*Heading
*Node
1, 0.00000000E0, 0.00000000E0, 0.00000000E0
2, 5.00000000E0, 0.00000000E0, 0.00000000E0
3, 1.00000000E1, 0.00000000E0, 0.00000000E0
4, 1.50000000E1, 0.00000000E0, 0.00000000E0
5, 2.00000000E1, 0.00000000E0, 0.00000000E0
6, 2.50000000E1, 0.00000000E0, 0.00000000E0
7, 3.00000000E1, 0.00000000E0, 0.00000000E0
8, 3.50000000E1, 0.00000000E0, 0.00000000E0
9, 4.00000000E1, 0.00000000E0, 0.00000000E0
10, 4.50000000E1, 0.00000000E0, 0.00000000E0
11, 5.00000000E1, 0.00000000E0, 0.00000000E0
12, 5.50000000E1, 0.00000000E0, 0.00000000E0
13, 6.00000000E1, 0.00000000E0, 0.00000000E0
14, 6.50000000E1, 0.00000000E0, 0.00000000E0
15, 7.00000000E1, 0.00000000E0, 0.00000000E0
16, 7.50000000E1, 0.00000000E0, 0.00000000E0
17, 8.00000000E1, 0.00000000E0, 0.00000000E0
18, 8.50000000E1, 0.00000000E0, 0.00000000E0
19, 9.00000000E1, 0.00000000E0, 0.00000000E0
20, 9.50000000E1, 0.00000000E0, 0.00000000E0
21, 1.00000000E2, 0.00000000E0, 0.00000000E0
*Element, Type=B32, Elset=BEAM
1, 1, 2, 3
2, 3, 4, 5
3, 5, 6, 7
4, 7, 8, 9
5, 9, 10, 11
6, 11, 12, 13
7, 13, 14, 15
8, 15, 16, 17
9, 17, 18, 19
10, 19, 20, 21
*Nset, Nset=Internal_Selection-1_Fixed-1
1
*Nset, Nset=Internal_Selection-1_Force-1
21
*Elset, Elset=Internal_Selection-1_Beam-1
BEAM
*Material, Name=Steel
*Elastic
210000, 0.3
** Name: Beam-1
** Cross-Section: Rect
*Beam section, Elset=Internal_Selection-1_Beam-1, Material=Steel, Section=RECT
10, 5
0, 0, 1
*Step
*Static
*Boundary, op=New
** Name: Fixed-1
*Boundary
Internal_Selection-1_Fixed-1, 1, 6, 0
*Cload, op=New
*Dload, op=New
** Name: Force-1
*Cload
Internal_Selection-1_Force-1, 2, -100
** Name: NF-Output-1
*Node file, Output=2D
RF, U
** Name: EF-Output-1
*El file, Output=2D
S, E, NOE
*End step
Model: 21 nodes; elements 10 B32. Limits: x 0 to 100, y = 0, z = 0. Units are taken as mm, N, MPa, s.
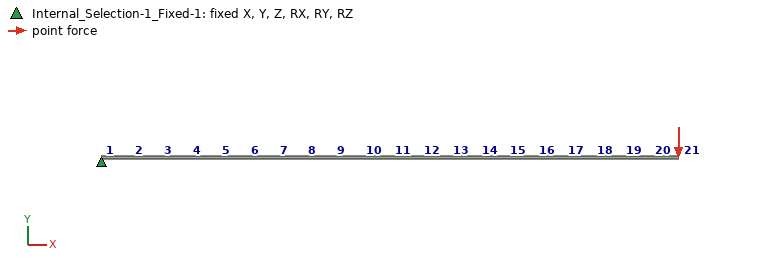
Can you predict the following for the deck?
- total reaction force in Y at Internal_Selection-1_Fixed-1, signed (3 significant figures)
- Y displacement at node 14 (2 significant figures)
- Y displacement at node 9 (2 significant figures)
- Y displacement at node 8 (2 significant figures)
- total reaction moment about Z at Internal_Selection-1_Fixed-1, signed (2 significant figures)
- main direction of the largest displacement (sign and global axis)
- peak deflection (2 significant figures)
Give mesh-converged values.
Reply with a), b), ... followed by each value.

a) 100 N
b) -0.76 mm
c) -0.32 mm
d) -0.25 mm
e) 10000 N·mm
f) -Y
g) 1.5 mm
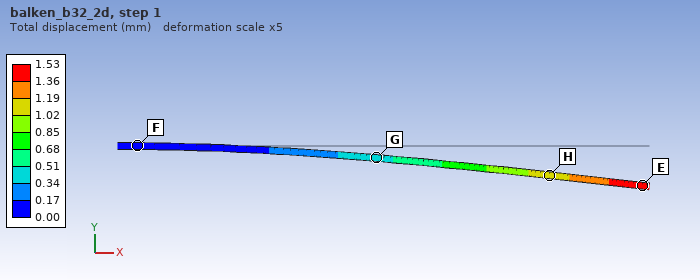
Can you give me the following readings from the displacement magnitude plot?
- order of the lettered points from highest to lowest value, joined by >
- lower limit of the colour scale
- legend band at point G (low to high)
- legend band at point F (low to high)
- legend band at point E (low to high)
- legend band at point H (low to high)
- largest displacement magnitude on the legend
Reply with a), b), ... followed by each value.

a) E > H > G > F
b) 0.00 mm
c) 0.34 to 0.51 mm
d) 0.00 to 0.17 mm
e) 1.36 to 1.53 mm
f) 1.02 to 1.19 mm
g) 1.53 mm
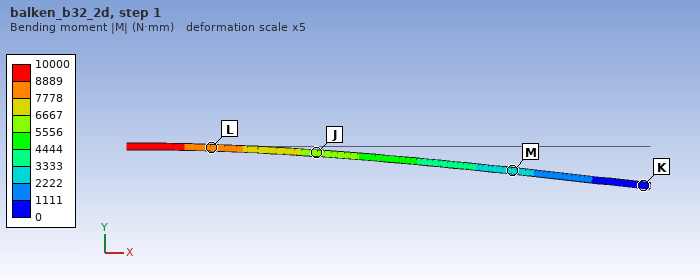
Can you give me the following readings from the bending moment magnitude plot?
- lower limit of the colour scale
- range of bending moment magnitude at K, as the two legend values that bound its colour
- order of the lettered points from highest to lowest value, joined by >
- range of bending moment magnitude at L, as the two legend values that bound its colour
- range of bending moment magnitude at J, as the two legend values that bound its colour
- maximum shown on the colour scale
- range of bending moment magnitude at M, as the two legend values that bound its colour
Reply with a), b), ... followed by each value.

a) 0 N·mm
b) 0 to 1111 N·mm
c) L > J > M > K
d) 7778 to 8889 N·mm
e) 5556 to 6667 N·mm
f) 10000 N·mm
g) 2222 to 3333 N·mm
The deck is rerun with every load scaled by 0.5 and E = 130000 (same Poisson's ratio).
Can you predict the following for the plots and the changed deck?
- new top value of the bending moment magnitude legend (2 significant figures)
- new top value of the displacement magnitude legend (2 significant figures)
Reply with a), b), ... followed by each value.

a) 5000 N·mm
b) 1.2 mm
